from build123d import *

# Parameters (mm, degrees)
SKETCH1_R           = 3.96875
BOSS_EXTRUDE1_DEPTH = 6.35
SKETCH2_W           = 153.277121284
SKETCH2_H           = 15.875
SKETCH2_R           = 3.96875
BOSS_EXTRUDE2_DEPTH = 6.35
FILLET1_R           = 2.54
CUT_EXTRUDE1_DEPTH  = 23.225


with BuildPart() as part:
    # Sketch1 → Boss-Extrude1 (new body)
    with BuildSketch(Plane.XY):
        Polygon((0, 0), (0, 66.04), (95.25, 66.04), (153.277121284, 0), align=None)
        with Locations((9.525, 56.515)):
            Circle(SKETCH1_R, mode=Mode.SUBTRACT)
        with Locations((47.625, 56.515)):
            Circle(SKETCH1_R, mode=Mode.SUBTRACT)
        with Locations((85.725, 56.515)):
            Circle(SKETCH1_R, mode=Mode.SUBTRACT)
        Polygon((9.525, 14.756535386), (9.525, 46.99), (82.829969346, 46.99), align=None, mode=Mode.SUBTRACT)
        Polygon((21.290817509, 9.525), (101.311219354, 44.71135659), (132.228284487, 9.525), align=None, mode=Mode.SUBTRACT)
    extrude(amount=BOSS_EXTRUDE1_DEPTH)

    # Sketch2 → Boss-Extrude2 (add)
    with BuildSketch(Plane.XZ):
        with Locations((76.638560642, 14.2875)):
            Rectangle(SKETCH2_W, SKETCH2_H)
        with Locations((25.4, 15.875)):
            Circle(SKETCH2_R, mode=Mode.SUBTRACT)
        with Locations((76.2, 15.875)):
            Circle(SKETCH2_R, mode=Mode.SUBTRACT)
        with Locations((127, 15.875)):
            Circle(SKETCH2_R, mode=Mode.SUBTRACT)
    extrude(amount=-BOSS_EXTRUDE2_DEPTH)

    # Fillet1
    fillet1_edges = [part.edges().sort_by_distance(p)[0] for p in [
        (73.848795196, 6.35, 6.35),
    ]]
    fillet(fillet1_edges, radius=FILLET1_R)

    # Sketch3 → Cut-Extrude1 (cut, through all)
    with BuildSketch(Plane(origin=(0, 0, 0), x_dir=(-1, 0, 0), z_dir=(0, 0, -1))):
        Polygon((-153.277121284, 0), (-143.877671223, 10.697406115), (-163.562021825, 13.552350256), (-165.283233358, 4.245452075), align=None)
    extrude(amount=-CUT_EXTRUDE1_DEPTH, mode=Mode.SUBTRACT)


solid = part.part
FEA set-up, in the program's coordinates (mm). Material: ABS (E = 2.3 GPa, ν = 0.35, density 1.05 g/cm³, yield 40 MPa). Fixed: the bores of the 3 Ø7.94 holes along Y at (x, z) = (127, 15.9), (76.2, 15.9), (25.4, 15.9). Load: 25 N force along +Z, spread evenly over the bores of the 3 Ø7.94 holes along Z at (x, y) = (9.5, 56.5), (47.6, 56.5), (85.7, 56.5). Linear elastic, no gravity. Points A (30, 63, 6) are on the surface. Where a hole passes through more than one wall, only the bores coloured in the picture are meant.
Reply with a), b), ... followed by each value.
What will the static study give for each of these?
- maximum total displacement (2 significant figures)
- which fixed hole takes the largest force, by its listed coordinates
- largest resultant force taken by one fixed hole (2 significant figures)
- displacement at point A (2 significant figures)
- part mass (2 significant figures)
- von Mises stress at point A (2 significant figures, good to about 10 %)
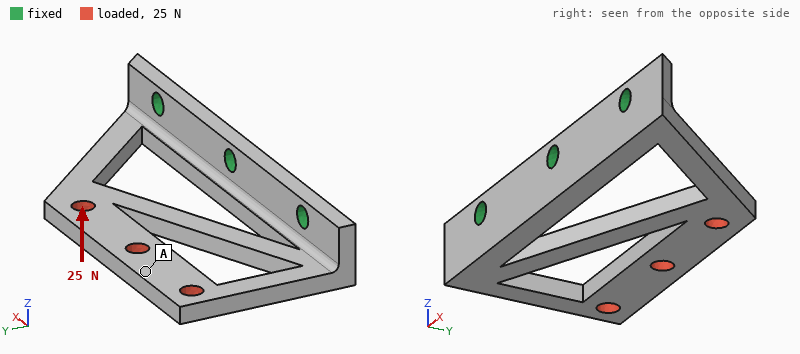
a) 1.9 mm
b) (25.4, 15.9)
c) 19 N
d) 1.7 mm
e) 48 g
f) 0.77 MPa
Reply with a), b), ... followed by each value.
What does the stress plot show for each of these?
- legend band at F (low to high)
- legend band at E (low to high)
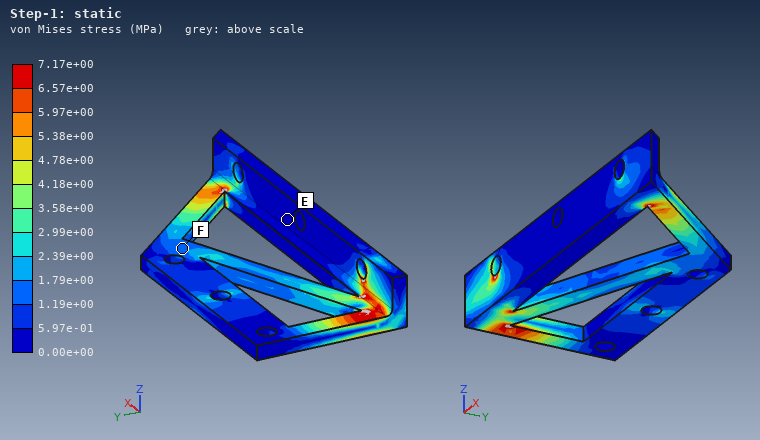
a) 1.19e+00 to 1.79e+00 MPa
b) 0.00e+00 to 5.97e-01 MPa
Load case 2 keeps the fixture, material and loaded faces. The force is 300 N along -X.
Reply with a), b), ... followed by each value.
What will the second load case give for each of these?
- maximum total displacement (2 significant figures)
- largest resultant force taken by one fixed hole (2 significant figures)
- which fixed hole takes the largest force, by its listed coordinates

a) 0.61 mm
b) 190 N
c) (25.4, 15.9)
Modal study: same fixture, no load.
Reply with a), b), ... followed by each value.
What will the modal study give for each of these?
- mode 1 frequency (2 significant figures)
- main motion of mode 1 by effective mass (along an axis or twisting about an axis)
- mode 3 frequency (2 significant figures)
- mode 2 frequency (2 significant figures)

a) 170 Hz
b) along Z
c) 860 Hz
d) 410 Hz
